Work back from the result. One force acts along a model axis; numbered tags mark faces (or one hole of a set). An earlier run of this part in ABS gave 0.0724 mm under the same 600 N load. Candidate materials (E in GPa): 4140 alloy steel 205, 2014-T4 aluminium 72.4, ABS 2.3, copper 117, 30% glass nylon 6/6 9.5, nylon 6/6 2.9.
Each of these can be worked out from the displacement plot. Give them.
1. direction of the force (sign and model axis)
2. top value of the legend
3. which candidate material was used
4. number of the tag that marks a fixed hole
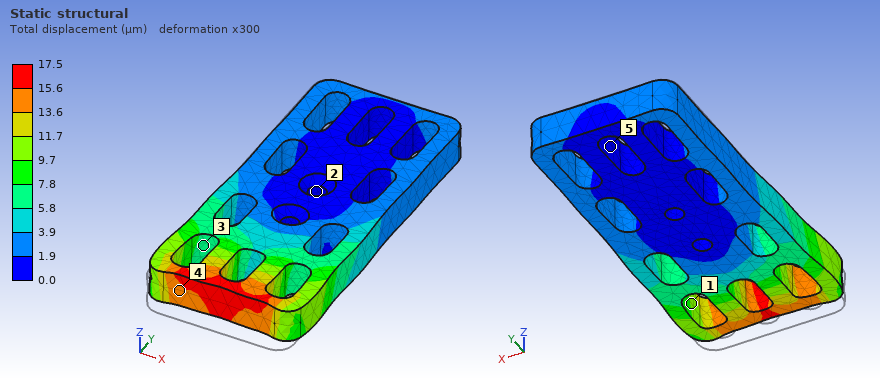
+Y
17.5 µm
30% glass nylon 6/6
2
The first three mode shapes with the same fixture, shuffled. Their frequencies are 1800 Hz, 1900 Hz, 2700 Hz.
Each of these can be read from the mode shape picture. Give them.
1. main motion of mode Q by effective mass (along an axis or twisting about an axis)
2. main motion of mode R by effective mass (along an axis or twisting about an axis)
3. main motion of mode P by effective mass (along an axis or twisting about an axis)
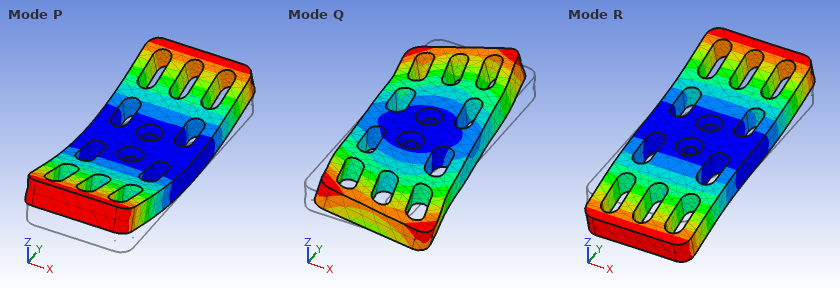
twisting about Z
twisting about X
along Z
